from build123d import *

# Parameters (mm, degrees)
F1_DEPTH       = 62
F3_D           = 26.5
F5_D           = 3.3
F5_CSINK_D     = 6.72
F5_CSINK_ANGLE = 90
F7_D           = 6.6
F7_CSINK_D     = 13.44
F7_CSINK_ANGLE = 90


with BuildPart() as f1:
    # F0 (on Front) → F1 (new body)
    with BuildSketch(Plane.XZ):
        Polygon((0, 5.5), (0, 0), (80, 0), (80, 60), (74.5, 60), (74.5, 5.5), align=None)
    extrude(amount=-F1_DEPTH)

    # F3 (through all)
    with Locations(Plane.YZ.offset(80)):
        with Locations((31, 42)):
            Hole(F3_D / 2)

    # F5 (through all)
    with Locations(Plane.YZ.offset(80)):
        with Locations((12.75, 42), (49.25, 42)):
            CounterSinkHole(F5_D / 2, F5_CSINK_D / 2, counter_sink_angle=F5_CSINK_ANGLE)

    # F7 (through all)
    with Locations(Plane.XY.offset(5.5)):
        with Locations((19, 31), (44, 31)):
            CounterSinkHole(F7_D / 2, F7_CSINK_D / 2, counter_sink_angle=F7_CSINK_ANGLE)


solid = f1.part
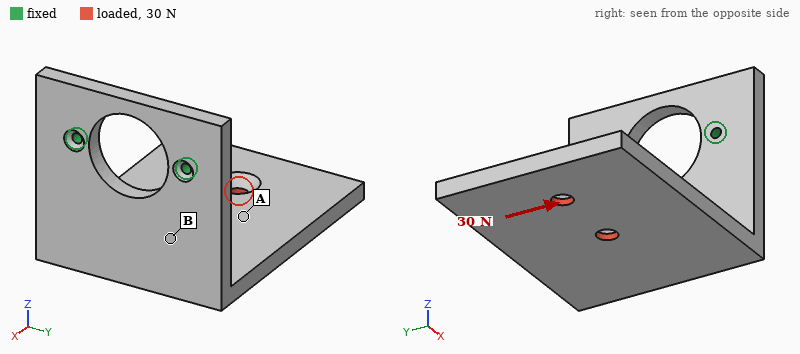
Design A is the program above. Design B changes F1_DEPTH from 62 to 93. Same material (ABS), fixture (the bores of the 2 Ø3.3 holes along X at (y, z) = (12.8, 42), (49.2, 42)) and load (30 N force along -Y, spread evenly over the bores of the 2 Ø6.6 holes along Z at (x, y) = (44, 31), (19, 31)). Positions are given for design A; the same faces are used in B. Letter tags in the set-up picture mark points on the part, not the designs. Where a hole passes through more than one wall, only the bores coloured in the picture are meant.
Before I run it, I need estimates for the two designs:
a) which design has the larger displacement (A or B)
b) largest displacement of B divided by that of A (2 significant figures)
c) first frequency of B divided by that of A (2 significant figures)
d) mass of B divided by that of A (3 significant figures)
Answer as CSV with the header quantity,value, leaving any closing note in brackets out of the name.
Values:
quantity,value
which design has the larger displacement,A
largest displacement of B divided by that of A,0.90
first frequency of B divided by that of A,0.92
mass of B divided by that of A,1.55
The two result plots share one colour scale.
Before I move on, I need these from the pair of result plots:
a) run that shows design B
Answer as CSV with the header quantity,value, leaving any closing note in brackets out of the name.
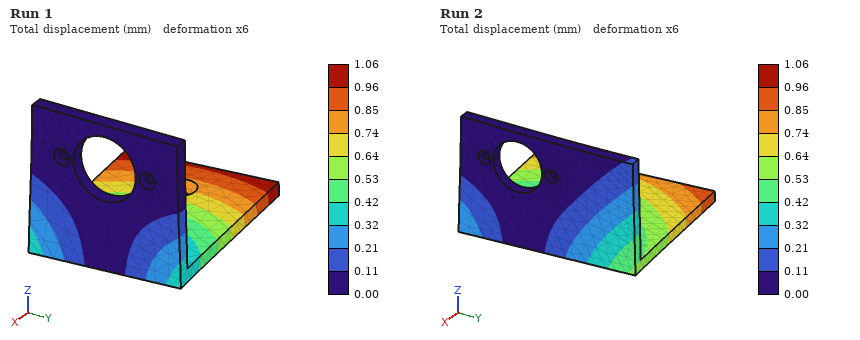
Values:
quantity,value
run that shows design B,Run 2
